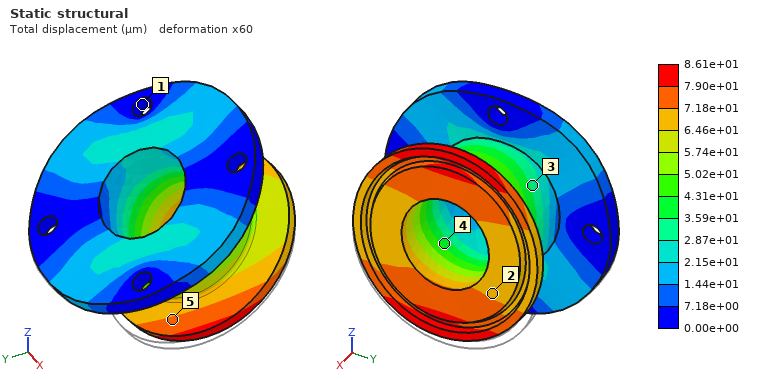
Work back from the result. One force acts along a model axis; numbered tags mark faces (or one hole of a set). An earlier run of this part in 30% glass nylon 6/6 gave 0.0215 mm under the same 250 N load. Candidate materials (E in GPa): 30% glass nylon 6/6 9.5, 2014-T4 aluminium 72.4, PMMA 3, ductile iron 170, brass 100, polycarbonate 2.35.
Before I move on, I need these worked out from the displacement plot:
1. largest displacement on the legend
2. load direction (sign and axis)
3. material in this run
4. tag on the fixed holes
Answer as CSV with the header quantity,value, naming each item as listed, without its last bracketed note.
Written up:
quantity,value
largest displacement on the legend,8.61e+01 µm
load direction,+Z
material in this run,polycarbonate
tag on the fixed holes,1
